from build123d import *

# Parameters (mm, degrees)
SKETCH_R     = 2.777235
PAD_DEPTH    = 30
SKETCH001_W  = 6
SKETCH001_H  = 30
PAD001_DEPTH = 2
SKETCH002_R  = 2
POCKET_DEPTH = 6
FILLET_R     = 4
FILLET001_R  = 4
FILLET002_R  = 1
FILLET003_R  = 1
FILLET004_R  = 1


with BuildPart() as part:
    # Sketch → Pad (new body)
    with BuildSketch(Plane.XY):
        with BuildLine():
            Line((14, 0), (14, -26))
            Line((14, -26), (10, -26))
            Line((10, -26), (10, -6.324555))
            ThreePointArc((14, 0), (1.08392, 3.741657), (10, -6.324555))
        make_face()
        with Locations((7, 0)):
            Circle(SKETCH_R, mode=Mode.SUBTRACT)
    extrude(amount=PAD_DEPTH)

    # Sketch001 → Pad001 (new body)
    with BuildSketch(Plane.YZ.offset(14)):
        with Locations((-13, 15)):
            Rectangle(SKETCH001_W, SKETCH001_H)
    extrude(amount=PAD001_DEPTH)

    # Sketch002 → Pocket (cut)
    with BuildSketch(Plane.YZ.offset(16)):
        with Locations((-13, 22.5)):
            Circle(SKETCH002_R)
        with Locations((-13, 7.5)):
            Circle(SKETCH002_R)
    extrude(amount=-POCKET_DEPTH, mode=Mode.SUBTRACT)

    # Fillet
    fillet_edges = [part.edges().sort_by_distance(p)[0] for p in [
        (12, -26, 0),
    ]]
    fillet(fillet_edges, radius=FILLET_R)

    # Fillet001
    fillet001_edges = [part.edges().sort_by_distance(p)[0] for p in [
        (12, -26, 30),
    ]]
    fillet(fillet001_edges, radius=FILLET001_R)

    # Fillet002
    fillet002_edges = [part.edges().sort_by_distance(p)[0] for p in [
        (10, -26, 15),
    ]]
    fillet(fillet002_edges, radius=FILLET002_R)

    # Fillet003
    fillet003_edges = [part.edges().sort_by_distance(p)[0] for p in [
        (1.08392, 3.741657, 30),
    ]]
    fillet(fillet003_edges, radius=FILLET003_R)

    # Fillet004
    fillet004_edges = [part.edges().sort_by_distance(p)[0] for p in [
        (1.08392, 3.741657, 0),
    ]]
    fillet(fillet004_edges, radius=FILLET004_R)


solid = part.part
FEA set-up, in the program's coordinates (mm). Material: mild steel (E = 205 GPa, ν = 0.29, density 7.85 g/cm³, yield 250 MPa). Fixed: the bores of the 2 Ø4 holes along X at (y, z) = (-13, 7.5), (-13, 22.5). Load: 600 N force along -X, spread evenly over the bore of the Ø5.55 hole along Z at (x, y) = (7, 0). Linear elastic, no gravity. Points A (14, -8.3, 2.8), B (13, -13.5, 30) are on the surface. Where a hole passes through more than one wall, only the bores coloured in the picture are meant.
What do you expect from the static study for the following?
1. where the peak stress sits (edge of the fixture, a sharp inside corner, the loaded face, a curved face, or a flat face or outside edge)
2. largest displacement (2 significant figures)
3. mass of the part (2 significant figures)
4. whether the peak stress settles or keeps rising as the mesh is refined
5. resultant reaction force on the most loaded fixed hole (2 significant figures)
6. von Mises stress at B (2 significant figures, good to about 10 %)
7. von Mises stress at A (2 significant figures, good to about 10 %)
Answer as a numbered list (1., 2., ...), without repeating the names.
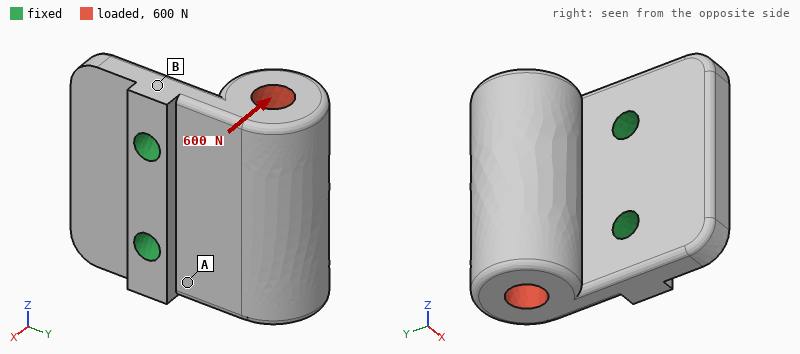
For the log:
1. edge of the fixture
2. 19 µm
3. 52 g
4. keeps rising
5. 300 N
6. 14 MPa
7. 55 MPa
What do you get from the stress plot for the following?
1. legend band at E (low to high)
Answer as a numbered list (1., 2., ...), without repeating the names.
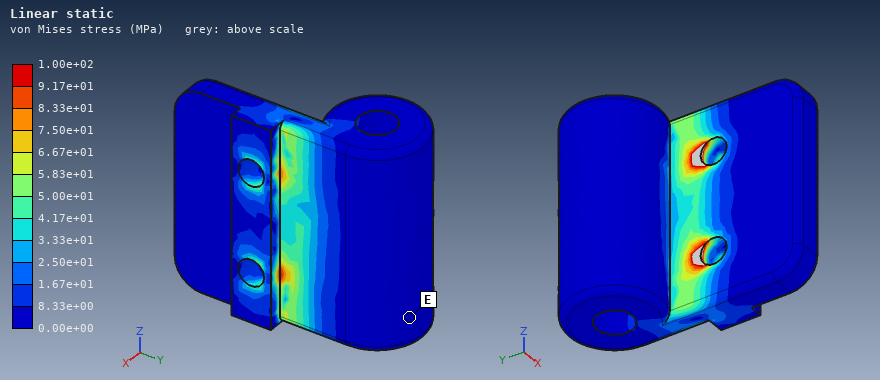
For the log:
1. 0.00e+00 to 8.33e+00 MPa
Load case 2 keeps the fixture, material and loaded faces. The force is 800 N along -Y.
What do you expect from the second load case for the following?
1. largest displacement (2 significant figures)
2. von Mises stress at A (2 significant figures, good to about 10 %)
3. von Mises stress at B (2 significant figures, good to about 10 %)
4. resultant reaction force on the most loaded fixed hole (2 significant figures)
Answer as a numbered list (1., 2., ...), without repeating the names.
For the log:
1. 15 µm
2. 39 MPa
3. 8.4 MPa
4. 400 N
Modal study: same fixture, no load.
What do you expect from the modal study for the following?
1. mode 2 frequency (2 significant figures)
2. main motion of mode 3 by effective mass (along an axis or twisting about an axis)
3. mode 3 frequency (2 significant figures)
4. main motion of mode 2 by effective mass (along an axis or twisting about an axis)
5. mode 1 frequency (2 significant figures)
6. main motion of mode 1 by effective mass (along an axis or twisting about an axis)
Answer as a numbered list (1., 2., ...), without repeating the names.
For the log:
1. 14 kHz
2. along Z
3. 20 kHz
4. along Z
5. 5400 Hz
6. along X
